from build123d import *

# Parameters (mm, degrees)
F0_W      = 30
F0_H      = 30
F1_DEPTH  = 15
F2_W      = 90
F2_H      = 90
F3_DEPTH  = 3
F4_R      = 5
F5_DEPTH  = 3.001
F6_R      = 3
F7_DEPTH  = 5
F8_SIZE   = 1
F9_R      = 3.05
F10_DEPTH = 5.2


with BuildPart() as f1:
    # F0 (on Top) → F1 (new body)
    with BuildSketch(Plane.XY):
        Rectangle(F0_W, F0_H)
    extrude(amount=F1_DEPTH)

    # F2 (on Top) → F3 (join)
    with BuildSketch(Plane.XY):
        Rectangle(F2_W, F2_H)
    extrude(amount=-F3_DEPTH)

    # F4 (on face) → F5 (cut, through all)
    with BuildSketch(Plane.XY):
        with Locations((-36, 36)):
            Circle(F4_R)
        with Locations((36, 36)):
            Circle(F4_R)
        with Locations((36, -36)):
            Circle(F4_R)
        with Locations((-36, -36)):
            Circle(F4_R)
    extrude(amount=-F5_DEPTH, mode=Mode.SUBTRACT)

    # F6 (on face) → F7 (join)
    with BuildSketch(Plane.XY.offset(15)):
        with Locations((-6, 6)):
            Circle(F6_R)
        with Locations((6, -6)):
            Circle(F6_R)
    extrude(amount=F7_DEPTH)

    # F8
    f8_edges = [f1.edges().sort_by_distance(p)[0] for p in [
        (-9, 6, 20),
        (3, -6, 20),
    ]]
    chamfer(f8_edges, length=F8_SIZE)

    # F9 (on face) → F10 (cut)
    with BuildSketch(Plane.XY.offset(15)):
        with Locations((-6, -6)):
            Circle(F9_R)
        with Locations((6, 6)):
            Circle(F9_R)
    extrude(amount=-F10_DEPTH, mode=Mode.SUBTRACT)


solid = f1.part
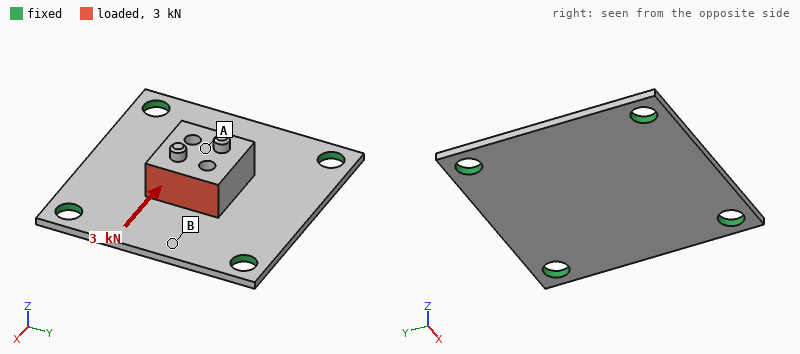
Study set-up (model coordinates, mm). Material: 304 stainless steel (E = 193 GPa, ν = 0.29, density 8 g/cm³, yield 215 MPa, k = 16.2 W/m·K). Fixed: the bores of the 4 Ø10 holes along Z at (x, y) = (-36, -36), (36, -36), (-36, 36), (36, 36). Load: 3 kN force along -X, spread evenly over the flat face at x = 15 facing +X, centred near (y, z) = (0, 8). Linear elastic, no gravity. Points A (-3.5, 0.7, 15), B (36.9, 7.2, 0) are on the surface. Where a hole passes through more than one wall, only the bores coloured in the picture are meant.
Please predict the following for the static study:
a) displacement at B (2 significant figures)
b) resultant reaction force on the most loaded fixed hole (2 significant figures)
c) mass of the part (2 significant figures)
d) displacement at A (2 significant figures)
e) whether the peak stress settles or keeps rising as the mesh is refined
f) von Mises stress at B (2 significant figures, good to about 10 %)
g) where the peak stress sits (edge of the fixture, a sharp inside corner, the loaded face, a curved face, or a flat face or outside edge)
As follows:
23 µm
880 N
290 g
31 µm
keeps rising
20 MPa
edge of the fixture
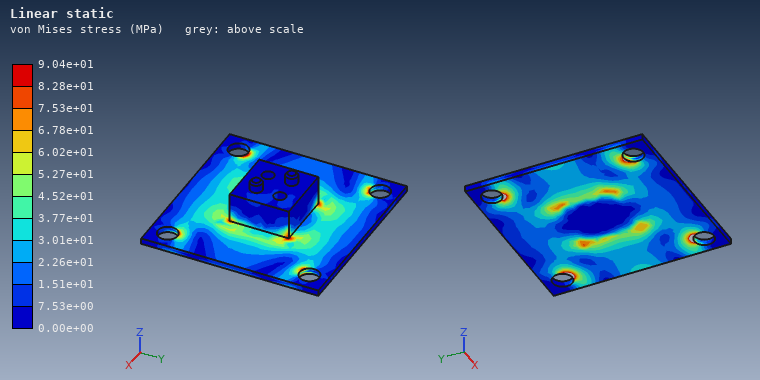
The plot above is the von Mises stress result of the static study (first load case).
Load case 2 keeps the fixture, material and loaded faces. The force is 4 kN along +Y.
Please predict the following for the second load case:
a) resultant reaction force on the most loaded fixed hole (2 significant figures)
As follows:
1.3 kN
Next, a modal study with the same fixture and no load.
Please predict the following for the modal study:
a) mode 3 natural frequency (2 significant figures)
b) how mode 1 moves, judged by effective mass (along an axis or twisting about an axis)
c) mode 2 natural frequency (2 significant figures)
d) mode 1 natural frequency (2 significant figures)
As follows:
3300 Hz
along Z
3300 Hz
1800 Hz
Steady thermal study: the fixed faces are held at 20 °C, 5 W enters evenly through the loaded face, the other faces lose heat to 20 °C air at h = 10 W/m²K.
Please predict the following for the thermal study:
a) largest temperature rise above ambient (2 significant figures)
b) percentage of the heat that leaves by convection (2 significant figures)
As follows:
28 K
37 %
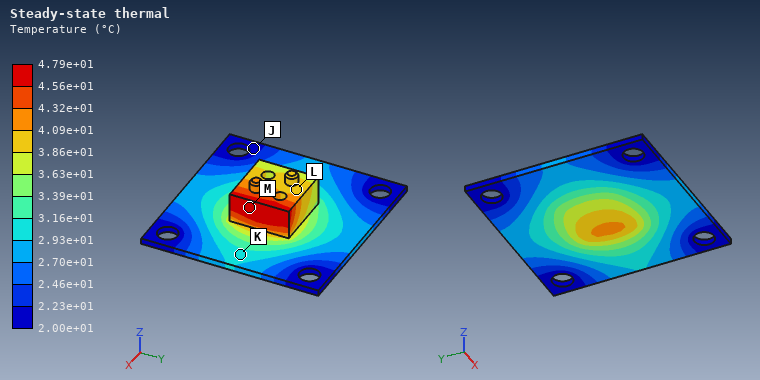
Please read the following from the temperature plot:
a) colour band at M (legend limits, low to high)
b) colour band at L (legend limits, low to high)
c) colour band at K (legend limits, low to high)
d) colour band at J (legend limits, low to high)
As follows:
4.56e+01 to 4.79e+01 °C
3.86e+01 to 4.09e+01 °C
2.93e+01 to 3.16e+01 °C
2.00e+01 to 2.23e+01 °C
